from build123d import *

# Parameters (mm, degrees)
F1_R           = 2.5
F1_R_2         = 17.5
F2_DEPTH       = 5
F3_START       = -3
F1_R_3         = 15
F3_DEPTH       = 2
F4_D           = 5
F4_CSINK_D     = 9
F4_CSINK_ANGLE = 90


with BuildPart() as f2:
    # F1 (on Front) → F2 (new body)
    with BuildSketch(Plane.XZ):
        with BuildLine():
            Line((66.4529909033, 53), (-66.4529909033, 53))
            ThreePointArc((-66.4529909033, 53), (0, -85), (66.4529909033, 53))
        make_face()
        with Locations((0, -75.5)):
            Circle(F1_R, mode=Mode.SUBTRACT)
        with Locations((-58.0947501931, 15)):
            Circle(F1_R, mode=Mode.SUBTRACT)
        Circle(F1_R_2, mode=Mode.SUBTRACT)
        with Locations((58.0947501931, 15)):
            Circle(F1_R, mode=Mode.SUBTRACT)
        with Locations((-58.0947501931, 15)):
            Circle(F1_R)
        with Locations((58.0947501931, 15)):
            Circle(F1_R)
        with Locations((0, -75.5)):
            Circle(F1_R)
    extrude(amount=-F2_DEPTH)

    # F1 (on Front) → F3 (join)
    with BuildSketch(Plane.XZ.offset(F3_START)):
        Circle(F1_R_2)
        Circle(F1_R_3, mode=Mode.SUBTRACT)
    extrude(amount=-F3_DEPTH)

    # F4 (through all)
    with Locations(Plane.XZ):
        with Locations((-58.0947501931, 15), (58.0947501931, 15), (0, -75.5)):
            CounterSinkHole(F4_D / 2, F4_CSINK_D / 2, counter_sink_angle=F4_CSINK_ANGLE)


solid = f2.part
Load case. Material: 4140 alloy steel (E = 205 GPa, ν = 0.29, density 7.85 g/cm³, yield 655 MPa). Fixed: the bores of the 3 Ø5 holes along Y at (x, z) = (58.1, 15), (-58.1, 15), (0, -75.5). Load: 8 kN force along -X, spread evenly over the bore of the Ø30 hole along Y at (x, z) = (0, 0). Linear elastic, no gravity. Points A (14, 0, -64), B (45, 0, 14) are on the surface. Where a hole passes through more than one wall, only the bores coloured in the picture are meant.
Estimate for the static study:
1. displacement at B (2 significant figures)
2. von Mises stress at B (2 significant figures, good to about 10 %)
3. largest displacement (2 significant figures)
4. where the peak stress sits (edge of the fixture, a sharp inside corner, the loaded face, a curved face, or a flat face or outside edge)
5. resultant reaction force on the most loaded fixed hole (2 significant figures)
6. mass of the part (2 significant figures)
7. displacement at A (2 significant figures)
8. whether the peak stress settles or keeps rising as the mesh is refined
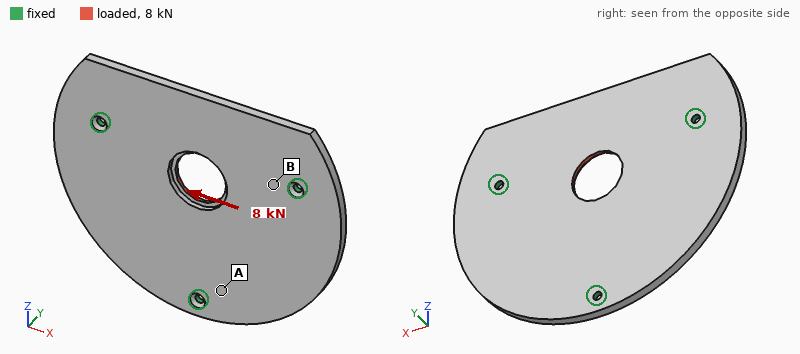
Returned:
3.9 µm
18 MPa
7.2 µm
edge of the fixture
3.2 kN
740 g
1.8 µm
keeps rising
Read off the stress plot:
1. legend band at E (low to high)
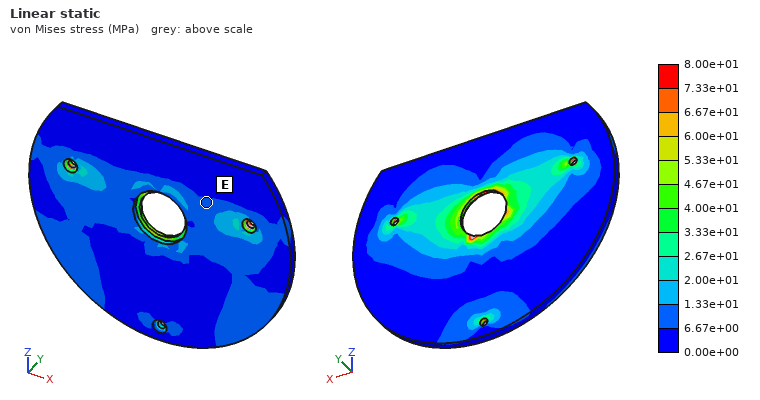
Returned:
6.67e+00 to 1.33e+01 MPa
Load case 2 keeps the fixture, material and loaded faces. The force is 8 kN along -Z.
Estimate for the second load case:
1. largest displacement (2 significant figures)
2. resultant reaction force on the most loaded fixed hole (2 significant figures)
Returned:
24 µm
2.8 kN
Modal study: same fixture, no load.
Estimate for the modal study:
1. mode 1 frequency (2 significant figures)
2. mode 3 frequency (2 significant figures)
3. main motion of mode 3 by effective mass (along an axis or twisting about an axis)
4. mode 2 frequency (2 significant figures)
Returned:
1200 Hz
1500 Hz
along Y
1300 Hz
